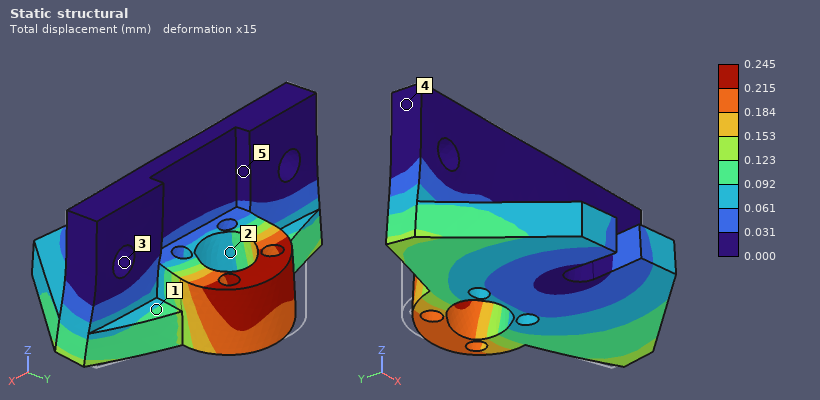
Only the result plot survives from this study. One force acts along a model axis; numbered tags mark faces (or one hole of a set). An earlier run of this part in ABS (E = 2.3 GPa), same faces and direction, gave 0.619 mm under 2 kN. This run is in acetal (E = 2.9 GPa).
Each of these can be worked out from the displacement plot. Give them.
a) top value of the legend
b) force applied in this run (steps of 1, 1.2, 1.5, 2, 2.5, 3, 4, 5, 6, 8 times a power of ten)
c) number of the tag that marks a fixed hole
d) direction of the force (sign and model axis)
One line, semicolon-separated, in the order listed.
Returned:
0.245 mm; 1 kN; 3; +X
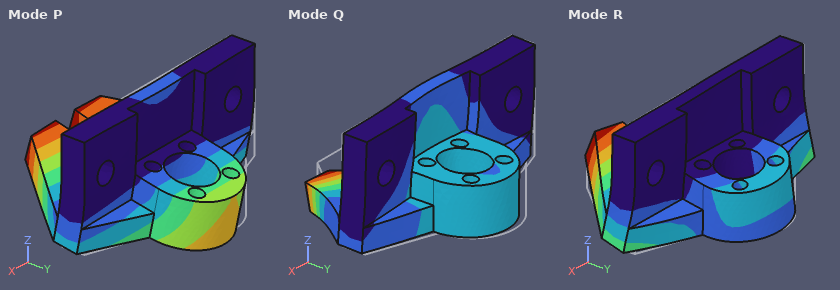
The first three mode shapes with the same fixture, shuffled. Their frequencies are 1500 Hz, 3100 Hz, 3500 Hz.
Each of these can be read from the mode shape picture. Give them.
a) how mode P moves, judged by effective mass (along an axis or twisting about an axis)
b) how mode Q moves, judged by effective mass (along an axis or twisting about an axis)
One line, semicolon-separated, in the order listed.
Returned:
along Y; along Y
